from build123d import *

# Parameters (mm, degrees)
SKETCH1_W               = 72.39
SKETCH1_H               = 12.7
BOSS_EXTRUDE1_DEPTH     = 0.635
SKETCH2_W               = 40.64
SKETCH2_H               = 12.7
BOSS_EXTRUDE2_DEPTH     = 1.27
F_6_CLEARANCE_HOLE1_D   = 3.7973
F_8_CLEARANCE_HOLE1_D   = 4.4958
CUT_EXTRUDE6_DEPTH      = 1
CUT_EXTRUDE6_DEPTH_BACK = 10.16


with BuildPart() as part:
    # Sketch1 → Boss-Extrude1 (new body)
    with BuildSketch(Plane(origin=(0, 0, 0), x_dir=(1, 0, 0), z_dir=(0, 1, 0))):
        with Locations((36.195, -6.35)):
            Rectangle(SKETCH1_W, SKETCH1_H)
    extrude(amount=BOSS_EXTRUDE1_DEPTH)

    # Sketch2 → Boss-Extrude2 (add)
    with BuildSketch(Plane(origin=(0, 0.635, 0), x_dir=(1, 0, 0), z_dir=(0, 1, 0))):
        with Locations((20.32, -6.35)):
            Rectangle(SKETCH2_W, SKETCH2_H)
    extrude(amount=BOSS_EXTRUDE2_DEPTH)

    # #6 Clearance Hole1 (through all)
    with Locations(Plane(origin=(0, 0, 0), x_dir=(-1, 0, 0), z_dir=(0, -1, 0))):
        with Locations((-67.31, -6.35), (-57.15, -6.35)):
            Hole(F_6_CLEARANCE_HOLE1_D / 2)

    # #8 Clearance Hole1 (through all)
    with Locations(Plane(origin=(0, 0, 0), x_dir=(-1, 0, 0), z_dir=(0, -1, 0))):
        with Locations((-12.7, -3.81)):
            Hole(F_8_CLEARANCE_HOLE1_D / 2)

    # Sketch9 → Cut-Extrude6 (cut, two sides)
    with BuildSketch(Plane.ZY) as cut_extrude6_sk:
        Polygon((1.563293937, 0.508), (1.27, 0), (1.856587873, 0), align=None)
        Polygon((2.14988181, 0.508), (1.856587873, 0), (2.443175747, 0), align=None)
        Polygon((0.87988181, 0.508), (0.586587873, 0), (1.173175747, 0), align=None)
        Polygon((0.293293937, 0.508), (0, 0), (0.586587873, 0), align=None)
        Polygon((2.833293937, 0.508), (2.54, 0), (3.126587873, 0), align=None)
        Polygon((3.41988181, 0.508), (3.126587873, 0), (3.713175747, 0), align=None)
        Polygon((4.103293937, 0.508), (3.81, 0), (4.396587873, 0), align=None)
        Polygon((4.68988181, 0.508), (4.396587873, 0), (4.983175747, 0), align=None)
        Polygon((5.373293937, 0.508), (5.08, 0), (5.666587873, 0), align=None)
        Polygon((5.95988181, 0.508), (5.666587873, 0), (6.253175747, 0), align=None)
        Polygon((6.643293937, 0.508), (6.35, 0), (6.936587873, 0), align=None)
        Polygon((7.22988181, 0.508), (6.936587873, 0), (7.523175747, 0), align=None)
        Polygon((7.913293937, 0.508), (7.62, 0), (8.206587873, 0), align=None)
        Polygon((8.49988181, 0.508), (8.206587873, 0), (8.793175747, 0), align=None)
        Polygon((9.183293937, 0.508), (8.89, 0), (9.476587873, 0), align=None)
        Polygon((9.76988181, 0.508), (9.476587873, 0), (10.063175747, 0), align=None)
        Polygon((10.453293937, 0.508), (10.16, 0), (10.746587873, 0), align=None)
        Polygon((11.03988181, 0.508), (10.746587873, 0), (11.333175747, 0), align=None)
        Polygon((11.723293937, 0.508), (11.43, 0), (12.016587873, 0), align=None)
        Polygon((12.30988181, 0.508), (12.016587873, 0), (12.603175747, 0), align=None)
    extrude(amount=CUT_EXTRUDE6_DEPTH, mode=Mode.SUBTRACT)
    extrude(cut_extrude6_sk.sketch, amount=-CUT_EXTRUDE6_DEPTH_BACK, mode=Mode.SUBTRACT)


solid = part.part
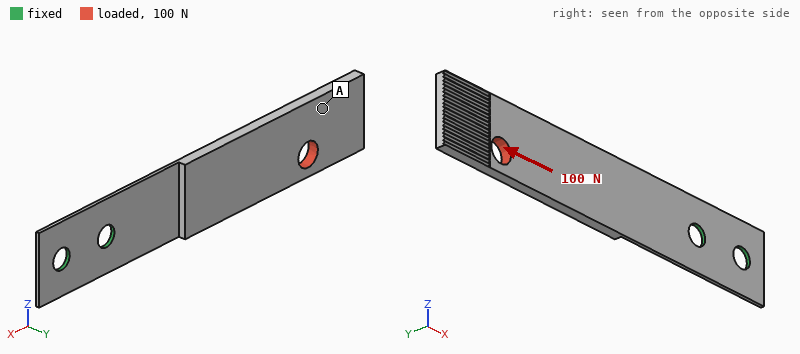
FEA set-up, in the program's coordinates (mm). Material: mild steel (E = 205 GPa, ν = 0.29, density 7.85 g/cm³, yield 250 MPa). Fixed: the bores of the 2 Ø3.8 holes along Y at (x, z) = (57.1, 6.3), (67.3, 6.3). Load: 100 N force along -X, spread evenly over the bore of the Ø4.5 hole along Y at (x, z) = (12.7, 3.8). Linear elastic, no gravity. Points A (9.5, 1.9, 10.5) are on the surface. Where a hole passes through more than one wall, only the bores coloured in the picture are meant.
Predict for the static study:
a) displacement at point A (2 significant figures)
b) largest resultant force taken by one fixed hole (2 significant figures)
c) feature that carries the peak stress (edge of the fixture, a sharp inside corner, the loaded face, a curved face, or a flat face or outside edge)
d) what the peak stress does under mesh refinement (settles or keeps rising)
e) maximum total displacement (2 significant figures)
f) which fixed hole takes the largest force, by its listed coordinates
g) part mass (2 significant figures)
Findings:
0.65 mm
88 N
edge of the fixture
keeps rising
0.82 mm
(57.1, 6.3)
9.1 g
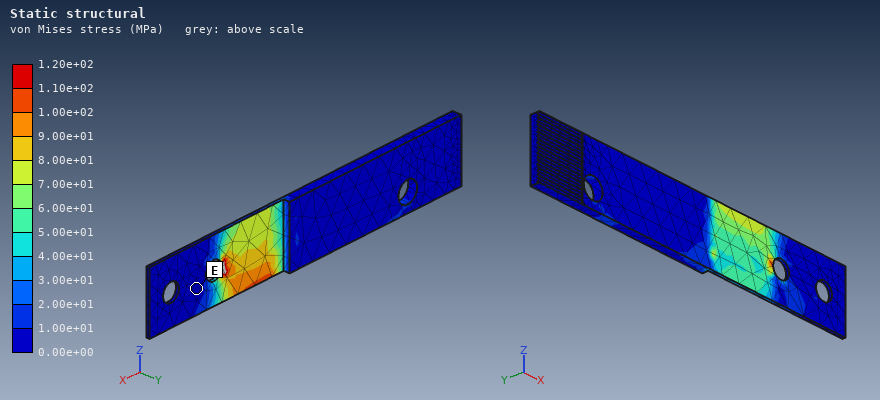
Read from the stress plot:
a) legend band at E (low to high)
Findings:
0.00e+00 to 1.00e+01 MPa
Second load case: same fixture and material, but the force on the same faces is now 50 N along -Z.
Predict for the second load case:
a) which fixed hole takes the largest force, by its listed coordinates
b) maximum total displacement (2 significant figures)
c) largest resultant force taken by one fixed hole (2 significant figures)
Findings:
(57.1, 6.3)
0.11 mm
160 N
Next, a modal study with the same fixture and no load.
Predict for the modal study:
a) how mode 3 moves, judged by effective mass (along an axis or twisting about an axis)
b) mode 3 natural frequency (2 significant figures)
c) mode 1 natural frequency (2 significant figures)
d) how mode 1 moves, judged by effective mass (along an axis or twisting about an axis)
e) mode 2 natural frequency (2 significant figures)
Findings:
along Y
1600 Hz
120 Hz
along Y
1300 Hz
